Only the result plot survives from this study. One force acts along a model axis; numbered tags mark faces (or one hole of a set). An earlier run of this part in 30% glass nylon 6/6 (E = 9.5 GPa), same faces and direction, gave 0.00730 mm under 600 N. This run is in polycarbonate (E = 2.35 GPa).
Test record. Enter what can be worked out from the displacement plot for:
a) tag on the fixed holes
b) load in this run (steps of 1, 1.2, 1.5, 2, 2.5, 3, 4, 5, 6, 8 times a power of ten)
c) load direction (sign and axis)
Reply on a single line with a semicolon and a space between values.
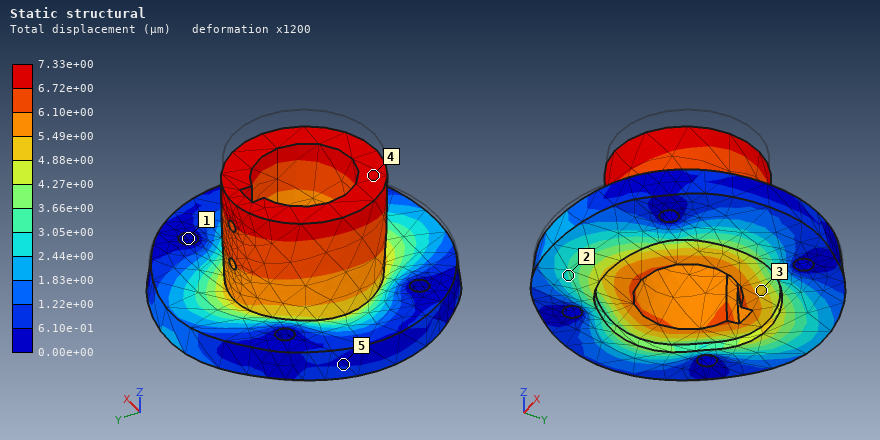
1; 150 N; -Z
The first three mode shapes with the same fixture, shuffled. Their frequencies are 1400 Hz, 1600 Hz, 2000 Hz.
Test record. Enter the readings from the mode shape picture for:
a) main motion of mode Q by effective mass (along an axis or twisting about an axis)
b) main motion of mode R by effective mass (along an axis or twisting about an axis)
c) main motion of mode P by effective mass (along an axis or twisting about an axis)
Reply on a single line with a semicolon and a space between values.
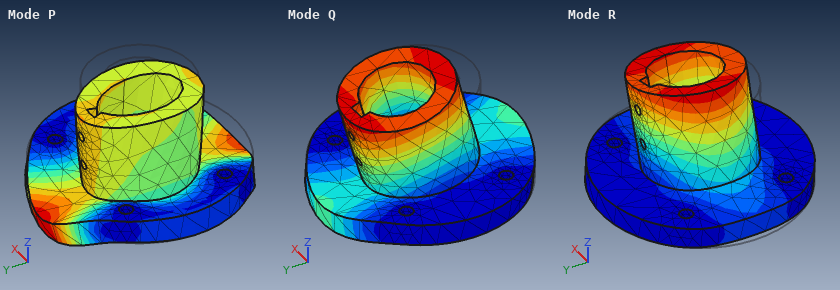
along Y; along X; along Z
